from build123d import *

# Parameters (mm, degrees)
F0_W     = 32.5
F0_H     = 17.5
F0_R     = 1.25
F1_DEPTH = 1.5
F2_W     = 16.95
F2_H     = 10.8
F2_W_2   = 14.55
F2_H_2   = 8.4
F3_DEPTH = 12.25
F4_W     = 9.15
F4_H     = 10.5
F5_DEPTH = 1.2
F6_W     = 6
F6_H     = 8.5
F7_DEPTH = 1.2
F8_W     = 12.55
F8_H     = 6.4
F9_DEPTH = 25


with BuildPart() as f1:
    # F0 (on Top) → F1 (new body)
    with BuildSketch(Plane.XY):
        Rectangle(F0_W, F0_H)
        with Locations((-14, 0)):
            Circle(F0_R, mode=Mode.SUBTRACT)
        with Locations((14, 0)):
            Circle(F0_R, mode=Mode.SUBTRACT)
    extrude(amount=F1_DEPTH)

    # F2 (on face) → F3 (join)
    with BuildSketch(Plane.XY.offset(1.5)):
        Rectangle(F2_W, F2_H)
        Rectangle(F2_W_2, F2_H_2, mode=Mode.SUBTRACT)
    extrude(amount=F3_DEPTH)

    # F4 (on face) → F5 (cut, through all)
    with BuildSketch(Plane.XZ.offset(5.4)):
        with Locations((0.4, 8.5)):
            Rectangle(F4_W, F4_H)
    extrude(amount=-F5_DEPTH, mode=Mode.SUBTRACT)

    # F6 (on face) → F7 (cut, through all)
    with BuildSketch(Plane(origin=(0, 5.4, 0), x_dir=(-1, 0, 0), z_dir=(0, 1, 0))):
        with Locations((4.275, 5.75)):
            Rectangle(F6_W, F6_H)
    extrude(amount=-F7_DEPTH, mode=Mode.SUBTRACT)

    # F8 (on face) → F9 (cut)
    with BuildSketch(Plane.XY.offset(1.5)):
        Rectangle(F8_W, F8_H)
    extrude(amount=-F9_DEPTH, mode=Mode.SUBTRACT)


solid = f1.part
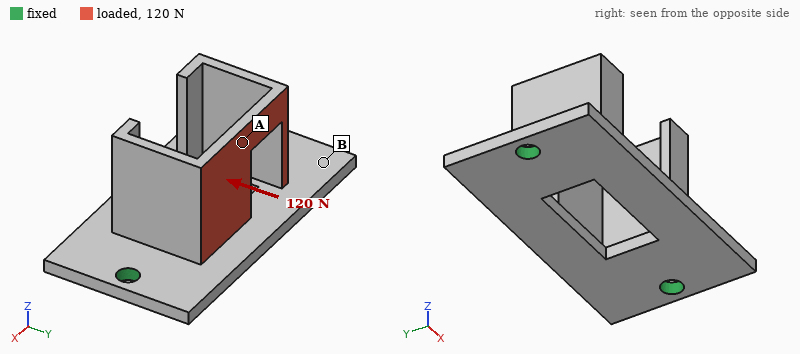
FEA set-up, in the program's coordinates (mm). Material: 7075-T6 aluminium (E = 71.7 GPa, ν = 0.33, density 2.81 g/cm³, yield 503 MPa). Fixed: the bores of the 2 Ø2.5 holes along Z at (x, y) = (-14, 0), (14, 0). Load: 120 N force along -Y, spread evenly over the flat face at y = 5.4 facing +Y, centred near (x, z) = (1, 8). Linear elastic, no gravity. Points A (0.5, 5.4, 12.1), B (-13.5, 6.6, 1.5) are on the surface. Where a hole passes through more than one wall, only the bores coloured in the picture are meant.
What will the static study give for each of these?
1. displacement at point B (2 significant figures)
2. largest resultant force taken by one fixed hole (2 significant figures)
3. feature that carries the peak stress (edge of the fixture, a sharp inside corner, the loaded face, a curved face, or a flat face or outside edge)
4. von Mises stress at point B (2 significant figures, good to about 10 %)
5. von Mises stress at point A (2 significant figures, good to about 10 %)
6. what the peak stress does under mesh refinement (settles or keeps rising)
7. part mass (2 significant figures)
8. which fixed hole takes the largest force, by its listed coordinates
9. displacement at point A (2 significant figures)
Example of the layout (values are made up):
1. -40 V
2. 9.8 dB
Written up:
1. 16 µm
2. 68 N
3. edge of the fixture
4. 15 MPa
5. 41 MPa
6. keeps rising
7. 3.6 g
8. (14, 0)
9. 85 µm
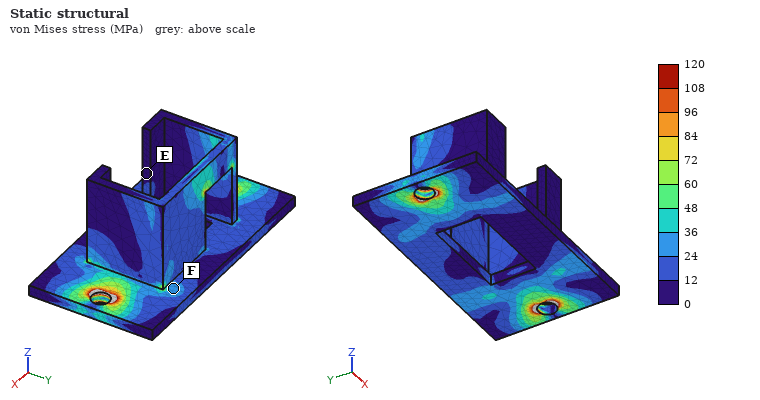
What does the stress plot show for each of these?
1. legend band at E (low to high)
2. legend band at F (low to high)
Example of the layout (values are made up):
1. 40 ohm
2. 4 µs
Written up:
1. 0 to 12 MPa
2. 24 to 36 MPa
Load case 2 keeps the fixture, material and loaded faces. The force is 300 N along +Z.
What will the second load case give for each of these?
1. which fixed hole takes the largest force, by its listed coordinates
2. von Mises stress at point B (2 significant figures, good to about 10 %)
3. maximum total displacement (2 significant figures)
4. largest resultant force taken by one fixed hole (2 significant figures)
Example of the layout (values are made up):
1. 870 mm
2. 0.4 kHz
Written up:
1. (14, 0)
2. 35 MPa
3. 0.16 mm
4. 180 N
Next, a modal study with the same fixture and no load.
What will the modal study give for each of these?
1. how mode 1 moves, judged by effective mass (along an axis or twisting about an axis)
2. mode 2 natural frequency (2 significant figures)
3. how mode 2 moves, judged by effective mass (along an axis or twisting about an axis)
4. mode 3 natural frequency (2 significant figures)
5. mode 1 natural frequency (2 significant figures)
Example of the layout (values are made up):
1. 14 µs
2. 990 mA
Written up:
1. along Y
2. 9400 Hz
3. along Z
4. 11 kHz
5. 5100 Hz
